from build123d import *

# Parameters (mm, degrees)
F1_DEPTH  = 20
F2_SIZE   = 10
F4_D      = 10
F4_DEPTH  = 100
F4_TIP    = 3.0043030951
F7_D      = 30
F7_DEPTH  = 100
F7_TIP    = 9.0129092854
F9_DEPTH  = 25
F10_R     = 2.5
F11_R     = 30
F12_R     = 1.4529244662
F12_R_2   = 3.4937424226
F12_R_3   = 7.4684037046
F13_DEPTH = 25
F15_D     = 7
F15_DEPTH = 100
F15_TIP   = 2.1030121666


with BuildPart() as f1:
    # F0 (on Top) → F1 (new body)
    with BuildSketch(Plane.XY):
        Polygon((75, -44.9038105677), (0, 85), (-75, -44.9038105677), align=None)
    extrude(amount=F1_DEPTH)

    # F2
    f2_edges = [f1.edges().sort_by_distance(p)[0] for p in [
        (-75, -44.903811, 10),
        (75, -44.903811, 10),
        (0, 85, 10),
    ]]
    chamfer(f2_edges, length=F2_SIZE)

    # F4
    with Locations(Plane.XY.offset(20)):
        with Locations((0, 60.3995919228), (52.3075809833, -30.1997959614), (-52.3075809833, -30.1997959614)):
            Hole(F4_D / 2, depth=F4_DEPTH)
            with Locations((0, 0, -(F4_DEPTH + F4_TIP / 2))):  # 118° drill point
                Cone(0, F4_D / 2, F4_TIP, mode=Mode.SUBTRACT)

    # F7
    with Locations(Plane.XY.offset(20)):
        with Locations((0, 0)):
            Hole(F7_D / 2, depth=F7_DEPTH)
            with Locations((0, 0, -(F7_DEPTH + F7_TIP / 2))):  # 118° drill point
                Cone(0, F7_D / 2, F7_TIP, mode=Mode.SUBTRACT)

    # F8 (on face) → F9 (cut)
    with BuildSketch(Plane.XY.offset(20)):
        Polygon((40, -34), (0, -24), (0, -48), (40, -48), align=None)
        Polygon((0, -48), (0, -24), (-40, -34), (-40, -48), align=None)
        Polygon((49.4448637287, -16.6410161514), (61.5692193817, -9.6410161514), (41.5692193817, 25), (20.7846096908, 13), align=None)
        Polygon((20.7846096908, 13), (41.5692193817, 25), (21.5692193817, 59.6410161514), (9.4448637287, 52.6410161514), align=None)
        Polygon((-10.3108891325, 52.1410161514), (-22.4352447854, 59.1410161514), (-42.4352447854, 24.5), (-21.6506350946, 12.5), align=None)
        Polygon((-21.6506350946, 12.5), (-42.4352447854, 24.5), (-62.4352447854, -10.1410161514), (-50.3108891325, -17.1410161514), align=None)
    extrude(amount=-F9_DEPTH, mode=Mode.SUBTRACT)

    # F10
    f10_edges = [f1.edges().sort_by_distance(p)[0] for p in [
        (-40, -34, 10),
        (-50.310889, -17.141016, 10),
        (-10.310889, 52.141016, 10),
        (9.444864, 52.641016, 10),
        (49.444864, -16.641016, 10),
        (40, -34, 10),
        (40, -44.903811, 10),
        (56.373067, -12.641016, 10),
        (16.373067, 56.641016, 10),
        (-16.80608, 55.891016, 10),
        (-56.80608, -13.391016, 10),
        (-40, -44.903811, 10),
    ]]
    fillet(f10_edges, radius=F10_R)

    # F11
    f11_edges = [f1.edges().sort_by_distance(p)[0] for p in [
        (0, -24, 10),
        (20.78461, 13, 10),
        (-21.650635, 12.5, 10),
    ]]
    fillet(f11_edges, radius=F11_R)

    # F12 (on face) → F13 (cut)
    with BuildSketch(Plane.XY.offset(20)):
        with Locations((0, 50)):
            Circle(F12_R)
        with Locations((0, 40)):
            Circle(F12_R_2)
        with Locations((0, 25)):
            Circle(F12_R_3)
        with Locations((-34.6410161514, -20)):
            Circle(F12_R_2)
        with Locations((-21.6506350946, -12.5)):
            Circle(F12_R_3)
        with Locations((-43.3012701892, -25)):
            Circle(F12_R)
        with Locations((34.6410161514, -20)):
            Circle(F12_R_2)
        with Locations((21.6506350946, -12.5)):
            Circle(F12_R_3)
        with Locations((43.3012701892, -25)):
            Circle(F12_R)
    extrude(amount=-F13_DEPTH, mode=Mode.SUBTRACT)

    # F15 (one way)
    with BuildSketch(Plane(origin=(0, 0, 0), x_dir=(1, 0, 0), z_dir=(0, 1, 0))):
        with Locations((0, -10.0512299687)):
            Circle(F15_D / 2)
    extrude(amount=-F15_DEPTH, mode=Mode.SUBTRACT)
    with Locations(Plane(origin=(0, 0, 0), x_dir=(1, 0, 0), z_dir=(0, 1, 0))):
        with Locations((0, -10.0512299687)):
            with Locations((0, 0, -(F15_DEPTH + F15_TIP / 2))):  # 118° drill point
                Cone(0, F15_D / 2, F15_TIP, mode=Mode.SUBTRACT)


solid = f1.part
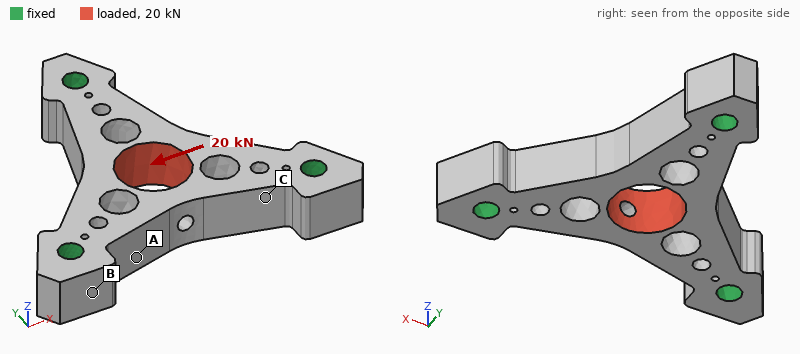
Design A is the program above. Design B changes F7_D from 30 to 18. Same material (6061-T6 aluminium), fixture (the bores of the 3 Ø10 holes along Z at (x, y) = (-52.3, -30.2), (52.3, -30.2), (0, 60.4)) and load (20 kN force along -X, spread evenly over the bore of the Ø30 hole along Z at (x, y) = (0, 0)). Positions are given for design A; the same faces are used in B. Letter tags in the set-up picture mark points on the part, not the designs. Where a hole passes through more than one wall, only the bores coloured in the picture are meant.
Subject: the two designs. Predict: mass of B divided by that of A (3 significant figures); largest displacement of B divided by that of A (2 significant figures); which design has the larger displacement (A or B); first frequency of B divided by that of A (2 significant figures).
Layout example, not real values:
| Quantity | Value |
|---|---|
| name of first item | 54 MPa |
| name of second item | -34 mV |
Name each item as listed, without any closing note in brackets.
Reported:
| Quantity | Value |
|---|---|
| mass of B divided by that of A | 1.09 |
| largest displacement of B divided by that of A | 0.69 |
| which design has the larger displacement | A |
| first frequency of B divided by that of A | 0.93 |
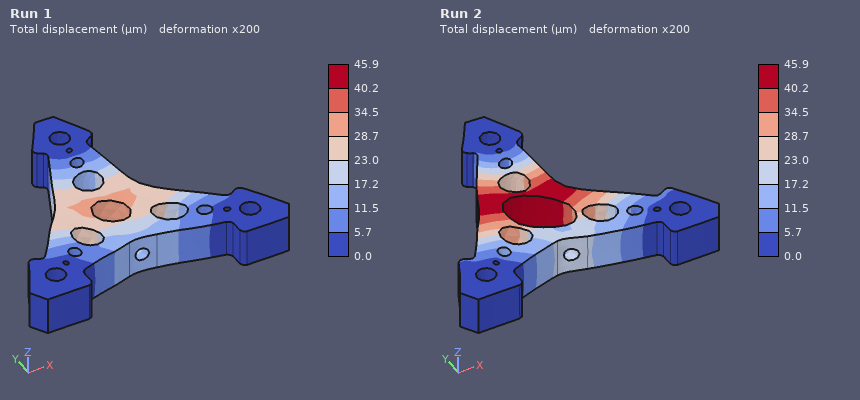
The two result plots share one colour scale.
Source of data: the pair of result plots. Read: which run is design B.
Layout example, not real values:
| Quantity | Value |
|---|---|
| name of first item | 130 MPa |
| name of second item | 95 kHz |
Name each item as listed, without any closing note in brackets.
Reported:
| Quantity | Value |
|---|---|
| which run is design B | Run 1 |
